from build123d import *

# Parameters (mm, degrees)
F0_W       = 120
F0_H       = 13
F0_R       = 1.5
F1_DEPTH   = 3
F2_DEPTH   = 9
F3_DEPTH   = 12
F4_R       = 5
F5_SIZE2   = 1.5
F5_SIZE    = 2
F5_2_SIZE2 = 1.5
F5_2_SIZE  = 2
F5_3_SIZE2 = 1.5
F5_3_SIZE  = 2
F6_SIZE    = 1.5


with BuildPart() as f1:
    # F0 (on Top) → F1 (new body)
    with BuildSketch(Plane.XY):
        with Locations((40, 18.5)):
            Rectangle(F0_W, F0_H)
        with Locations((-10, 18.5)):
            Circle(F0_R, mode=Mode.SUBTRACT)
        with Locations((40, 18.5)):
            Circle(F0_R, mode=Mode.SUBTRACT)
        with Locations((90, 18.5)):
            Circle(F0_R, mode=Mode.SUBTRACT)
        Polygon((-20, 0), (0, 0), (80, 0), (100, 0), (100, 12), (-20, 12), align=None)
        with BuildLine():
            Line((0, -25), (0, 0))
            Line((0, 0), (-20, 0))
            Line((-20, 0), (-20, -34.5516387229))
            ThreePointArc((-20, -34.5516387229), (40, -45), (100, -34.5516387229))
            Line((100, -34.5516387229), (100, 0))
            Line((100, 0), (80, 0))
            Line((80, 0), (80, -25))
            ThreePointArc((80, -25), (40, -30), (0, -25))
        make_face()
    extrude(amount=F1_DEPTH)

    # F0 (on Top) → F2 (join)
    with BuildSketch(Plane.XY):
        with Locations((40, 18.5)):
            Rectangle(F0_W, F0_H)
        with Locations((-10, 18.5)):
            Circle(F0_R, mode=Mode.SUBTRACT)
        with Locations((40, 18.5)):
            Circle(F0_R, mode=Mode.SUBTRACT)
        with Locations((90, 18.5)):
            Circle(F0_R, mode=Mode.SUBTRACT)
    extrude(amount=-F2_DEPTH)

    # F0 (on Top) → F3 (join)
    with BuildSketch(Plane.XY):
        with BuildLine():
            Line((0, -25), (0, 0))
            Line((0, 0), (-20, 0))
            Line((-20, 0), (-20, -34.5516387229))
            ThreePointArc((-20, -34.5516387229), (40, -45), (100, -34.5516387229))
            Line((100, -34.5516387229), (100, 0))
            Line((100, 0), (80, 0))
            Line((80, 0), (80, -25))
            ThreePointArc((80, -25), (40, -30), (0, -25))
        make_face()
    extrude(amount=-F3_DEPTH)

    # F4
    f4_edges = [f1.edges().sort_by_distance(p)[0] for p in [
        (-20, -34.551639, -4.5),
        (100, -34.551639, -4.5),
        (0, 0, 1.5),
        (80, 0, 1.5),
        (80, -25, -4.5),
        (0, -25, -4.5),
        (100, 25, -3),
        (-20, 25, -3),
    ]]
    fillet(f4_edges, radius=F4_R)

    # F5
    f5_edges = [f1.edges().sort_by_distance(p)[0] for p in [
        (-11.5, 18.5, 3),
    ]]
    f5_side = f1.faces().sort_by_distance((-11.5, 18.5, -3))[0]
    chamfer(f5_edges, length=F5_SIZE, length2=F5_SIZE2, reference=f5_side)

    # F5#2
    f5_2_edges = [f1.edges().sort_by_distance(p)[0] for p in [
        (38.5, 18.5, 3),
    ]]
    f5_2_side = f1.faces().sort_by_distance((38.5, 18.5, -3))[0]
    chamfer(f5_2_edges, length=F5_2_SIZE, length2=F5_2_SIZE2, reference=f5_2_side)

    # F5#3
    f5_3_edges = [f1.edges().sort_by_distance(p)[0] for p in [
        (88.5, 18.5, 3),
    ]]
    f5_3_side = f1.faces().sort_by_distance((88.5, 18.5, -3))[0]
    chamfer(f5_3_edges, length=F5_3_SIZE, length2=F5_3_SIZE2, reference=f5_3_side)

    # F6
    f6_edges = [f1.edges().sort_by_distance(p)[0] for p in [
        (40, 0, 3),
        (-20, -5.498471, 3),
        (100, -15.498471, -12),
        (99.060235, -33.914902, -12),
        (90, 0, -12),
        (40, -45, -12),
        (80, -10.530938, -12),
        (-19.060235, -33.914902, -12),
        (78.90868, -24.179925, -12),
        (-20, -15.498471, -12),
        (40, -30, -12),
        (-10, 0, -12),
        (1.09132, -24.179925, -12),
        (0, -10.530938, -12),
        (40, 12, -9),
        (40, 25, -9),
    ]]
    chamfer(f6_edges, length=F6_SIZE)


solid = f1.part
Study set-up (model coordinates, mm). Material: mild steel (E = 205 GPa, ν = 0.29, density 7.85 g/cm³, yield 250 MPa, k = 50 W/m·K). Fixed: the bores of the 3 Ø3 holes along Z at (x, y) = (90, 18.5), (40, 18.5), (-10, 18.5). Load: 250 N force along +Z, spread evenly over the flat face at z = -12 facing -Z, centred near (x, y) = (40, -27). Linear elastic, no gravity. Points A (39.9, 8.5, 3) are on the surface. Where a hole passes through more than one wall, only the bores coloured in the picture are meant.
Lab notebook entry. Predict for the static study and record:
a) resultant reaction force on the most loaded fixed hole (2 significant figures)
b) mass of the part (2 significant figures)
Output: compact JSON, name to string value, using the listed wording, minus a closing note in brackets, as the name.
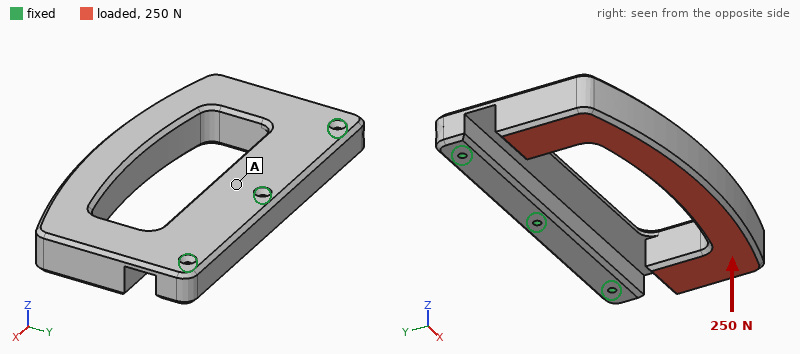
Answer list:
{"resultant reaction force on the most loaded fixed hole": "120 N", "mass of the part": "490 g"}
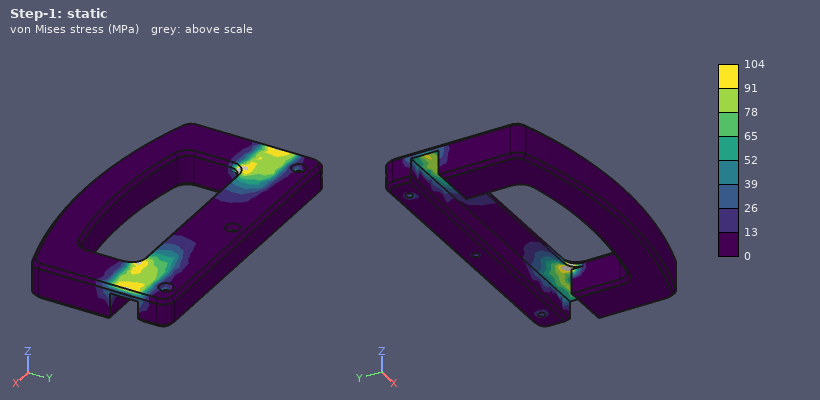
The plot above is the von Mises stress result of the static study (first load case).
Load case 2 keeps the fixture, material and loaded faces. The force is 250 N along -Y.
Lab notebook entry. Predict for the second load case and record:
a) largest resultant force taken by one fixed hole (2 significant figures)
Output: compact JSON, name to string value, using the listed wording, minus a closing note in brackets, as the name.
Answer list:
{"largest resultant force taken by one fixed hole": "130 N"}
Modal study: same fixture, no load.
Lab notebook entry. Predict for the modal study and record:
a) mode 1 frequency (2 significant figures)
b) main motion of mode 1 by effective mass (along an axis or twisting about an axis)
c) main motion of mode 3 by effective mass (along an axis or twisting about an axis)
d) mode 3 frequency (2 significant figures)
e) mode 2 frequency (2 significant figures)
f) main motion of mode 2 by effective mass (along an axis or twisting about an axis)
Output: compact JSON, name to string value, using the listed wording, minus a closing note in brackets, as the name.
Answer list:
{"mode 1 frequency": "330 Hz", "main motion of mode 1 by effective mass": "along Z", "main motion of mode 3 by effective mass": "along X", "mode 3 frequency": "2900 Hz", "mode 2 frequency": "1600 Hz", "main motion of mode 2 by effective mass": "twisting about Y"}
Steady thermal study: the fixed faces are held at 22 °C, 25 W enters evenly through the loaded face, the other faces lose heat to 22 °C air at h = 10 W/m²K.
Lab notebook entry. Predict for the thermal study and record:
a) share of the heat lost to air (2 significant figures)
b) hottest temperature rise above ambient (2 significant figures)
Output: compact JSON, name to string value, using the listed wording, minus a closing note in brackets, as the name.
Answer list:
{"share of the heat lost to air": "23 %", "hottest temperature rise above ambient": "76 K"}
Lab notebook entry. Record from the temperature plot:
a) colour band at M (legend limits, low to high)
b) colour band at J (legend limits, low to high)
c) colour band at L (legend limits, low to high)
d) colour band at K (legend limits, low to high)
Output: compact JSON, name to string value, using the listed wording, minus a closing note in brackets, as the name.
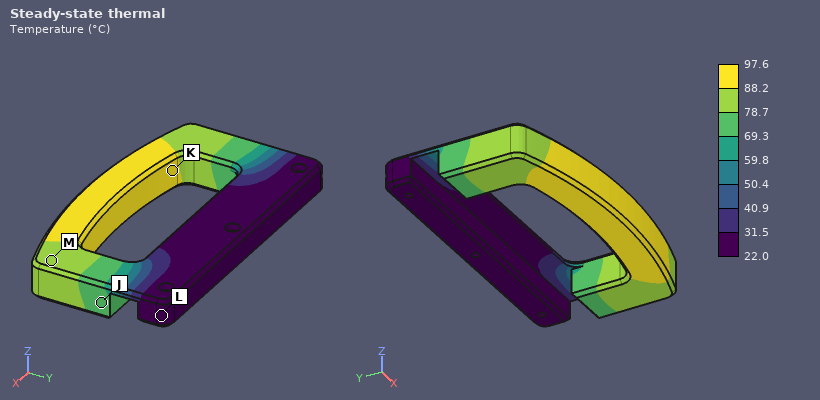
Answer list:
{"colour band at M": "78.7 to 88.2 °C", "colour band at J": "69.3 to 78.7 °C", "colour band at L": "22.0 to 31.5 °C", "colour band at K": "88.2 to 97.6 °C"}
